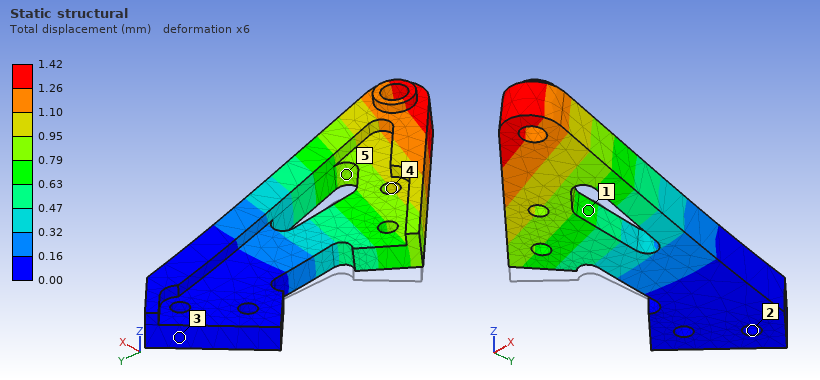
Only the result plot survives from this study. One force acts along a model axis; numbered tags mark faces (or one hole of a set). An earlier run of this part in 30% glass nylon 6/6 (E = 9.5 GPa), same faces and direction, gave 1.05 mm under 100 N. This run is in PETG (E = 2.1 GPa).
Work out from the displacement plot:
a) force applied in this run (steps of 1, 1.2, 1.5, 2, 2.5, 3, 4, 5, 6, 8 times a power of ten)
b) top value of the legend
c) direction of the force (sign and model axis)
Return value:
30 N
1.42 mm
+Z
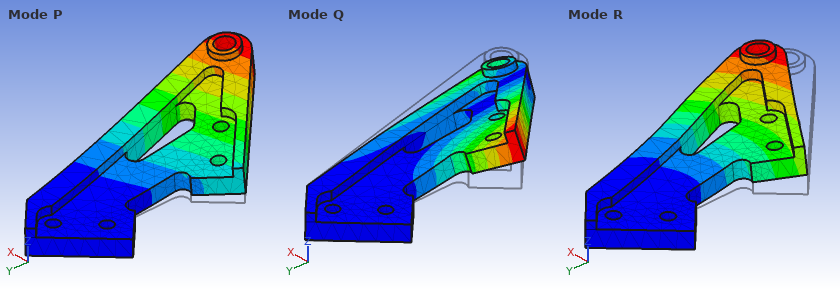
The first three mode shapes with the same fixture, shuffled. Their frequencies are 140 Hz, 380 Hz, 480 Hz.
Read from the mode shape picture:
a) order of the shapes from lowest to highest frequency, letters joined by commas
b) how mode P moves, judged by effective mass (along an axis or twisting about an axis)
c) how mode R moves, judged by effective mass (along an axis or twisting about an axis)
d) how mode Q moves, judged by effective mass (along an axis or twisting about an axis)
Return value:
P, R, Q
along Z
along X
twisting about Y
